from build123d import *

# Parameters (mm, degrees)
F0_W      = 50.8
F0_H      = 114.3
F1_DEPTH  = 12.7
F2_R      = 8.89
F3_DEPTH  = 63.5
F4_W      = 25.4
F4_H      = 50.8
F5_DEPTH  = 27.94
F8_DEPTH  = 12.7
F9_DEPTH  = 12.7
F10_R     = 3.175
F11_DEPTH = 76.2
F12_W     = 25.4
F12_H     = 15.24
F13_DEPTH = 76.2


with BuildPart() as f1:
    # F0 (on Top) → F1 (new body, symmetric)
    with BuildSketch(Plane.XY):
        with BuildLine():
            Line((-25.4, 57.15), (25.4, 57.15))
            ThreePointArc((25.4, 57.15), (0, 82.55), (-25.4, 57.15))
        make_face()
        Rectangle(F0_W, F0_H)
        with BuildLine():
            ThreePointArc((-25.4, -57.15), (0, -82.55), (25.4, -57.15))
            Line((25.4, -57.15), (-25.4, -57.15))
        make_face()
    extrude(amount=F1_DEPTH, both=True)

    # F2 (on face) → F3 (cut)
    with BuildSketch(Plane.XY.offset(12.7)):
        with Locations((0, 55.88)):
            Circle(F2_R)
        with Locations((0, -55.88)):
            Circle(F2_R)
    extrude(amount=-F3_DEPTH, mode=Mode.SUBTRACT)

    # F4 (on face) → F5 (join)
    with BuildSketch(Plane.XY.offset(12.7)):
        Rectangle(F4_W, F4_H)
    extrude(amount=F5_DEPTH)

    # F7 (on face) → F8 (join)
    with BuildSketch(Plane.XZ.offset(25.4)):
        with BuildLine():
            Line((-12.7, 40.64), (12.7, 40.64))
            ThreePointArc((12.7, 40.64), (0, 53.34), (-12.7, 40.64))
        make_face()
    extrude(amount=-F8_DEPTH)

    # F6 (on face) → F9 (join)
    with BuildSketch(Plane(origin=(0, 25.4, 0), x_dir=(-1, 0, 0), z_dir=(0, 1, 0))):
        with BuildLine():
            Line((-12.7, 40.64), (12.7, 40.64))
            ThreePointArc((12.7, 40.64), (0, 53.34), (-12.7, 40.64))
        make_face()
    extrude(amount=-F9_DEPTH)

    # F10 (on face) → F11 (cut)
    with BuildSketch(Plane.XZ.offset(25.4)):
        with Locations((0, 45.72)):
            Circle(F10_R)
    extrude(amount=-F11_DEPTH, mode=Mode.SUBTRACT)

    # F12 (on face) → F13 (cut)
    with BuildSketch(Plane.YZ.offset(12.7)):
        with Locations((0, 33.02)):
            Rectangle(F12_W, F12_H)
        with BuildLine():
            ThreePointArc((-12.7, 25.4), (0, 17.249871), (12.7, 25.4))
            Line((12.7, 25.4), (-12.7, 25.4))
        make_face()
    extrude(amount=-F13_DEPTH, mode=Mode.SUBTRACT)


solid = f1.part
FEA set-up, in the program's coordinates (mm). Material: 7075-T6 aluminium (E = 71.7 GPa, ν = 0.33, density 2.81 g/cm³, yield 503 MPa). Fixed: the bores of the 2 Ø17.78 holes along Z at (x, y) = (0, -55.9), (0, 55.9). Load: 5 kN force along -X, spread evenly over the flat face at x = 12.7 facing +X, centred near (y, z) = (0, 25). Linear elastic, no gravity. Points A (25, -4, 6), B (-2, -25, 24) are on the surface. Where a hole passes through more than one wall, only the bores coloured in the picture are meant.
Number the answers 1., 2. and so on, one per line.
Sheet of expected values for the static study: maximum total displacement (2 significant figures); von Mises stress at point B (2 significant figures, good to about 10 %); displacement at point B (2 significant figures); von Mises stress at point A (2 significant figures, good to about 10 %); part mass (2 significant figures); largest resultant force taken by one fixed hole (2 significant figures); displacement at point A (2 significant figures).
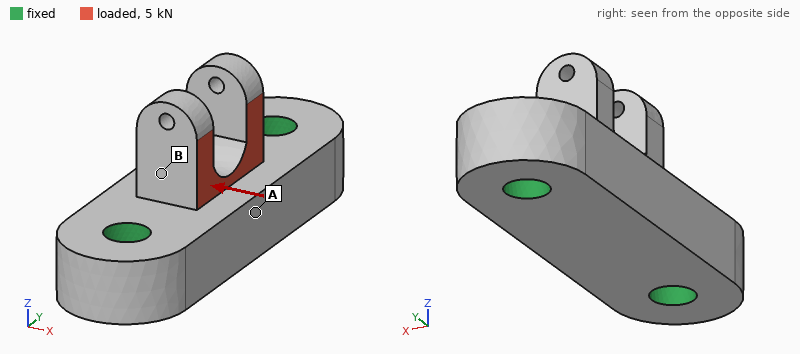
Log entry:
1. 37 µm
2. 8.8 MPa
3. 17 µm
4. 4.4 MPa
5. 600 g
6. 2.5 kN
7. 12 µm
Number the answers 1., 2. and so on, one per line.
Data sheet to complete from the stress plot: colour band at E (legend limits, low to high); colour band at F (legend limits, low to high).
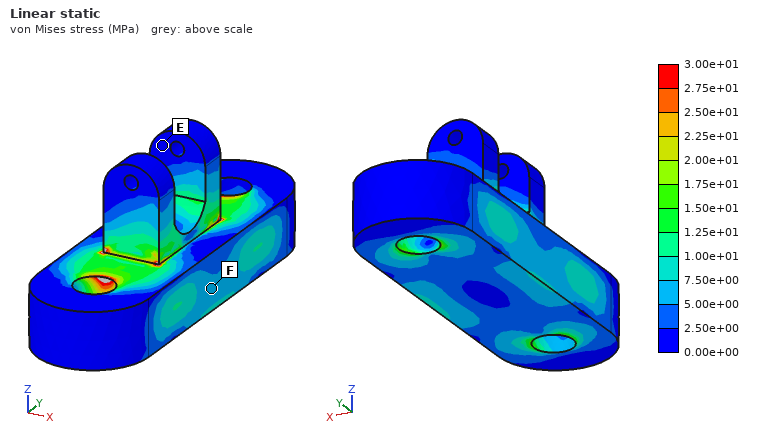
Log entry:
1. 0.00e+00 to 2.50e+00 MPa
2. 5.00e+00 to 7.50e+00 MPa
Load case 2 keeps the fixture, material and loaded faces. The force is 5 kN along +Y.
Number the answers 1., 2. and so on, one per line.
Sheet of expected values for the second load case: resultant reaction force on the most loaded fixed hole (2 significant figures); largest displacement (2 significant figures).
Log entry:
1. 2.9 kN
2. 29 µm
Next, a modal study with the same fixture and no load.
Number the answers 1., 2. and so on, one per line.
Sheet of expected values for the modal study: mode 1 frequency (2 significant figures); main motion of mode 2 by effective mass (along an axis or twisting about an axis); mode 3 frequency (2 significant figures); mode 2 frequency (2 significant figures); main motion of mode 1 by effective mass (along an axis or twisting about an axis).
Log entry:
1. 6400 Hz
2. along Z
3. 7900 Hz
4. 7500 Hz
5. along X
